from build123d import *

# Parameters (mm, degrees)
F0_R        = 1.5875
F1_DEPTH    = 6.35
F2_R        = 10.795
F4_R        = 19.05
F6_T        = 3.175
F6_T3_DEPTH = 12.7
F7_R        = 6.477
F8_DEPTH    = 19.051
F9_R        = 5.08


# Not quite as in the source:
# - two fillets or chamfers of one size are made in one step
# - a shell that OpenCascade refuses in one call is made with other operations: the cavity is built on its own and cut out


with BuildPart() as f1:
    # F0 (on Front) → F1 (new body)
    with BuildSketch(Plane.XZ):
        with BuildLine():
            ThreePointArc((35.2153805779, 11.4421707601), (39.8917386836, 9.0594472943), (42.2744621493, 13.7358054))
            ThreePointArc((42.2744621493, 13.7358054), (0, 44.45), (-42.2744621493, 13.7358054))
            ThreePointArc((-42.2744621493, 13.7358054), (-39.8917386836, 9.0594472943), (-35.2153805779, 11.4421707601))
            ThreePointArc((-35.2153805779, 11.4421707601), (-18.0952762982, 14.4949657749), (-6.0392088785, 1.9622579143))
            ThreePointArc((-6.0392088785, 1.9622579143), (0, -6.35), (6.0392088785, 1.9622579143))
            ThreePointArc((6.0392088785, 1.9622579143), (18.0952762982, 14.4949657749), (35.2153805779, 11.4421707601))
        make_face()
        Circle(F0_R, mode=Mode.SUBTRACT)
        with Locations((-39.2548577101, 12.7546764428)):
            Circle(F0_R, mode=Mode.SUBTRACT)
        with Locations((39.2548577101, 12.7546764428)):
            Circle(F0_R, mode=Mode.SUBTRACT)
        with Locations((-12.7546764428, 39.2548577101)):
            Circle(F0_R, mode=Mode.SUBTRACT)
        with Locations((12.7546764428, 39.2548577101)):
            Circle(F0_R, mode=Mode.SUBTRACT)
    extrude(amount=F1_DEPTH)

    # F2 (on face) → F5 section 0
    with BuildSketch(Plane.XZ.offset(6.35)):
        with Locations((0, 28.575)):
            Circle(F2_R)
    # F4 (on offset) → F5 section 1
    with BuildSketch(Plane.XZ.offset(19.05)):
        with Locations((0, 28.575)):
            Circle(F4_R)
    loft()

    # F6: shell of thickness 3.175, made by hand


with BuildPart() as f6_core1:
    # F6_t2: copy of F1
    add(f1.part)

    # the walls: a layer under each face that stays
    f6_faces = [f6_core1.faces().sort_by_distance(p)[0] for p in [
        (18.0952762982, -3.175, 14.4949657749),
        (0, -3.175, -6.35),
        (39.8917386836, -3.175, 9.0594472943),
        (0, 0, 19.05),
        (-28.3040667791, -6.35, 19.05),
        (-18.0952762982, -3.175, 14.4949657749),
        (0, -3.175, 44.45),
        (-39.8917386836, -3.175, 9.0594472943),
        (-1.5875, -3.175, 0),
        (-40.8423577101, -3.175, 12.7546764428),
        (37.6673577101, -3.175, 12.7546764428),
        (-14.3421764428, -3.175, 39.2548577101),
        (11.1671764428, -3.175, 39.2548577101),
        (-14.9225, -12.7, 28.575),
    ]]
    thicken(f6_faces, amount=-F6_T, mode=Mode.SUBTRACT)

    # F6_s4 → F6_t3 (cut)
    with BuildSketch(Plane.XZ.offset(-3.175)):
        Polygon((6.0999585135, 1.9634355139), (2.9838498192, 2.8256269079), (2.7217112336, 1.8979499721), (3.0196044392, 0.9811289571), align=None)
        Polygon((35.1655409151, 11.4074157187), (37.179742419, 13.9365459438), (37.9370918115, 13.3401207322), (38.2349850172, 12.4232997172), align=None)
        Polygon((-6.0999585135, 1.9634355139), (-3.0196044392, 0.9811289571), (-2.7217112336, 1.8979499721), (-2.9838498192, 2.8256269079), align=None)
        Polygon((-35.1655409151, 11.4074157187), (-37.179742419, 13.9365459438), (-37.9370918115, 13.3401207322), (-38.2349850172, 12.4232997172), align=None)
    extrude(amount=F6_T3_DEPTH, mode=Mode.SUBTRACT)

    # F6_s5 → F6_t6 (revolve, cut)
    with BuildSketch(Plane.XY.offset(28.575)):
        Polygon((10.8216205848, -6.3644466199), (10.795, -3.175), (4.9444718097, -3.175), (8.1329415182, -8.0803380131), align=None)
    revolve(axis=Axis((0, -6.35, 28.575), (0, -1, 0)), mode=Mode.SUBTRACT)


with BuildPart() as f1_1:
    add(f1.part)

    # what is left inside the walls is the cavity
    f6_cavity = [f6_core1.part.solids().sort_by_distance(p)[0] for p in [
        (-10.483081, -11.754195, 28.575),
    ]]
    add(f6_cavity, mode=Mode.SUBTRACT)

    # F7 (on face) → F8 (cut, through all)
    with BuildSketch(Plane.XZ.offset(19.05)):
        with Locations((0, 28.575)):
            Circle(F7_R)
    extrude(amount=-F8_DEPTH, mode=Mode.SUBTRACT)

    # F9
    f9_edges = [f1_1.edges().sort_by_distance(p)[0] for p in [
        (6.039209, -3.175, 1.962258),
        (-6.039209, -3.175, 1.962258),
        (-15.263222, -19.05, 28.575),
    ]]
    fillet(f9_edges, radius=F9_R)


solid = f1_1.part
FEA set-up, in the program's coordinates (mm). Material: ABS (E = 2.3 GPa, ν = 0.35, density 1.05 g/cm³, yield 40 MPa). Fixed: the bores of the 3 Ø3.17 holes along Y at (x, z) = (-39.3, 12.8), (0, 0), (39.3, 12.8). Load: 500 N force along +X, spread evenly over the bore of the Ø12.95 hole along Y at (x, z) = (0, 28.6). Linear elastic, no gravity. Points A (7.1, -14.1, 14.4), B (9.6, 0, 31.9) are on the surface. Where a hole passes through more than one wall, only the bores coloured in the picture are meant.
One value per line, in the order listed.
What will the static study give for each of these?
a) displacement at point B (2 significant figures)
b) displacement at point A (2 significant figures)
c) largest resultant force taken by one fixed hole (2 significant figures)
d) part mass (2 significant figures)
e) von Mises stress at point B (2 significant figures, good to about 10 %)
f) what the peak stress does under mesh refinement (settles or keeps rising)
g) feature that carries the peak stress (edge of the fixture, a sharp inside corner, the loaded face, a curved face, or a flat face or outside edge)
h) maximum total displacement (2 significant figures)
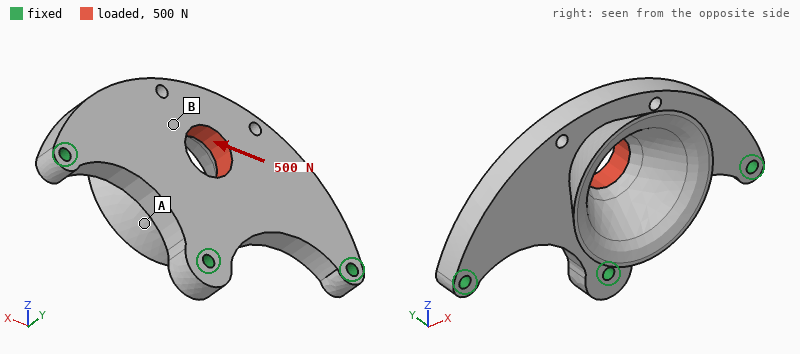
53 µm
38 µm
220 N
18 g
3.0 MPa
keeps rising
edge of the fixture
61 µm
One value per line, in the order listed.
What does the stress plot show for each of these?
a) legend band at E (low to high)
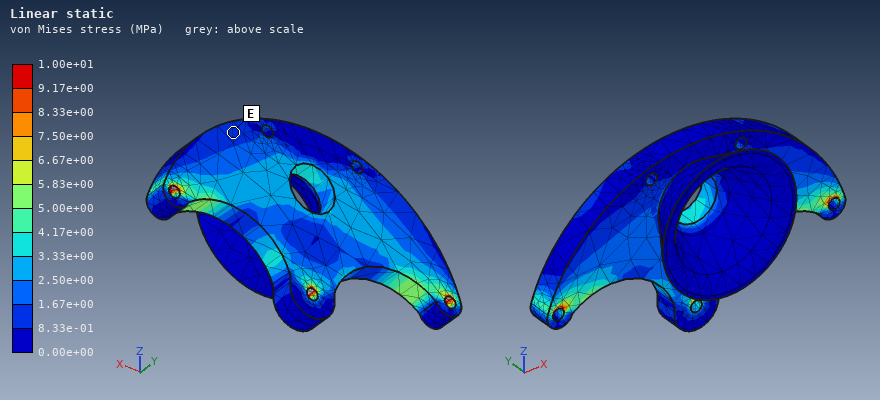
8.33e-01 to 1.67e+00 MPa
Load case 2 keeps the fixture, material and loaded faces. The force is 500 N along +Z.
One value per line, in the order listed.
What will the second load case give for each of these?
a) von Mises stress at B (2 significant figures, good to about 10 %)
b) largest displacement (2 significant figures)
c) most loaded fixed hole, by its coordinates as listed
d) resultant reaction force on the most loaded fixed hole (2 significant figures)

2.1 MPa
95 µm
(0, 0)
360 N
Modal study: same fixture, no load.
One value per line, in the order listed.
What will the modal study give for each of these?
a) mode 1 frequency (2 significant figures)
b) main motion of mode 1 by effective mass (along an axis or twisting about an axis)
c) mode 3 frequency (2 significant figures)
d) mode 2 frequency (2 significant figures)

710 Hz
along Y
2800 Hz
1900 Hz
